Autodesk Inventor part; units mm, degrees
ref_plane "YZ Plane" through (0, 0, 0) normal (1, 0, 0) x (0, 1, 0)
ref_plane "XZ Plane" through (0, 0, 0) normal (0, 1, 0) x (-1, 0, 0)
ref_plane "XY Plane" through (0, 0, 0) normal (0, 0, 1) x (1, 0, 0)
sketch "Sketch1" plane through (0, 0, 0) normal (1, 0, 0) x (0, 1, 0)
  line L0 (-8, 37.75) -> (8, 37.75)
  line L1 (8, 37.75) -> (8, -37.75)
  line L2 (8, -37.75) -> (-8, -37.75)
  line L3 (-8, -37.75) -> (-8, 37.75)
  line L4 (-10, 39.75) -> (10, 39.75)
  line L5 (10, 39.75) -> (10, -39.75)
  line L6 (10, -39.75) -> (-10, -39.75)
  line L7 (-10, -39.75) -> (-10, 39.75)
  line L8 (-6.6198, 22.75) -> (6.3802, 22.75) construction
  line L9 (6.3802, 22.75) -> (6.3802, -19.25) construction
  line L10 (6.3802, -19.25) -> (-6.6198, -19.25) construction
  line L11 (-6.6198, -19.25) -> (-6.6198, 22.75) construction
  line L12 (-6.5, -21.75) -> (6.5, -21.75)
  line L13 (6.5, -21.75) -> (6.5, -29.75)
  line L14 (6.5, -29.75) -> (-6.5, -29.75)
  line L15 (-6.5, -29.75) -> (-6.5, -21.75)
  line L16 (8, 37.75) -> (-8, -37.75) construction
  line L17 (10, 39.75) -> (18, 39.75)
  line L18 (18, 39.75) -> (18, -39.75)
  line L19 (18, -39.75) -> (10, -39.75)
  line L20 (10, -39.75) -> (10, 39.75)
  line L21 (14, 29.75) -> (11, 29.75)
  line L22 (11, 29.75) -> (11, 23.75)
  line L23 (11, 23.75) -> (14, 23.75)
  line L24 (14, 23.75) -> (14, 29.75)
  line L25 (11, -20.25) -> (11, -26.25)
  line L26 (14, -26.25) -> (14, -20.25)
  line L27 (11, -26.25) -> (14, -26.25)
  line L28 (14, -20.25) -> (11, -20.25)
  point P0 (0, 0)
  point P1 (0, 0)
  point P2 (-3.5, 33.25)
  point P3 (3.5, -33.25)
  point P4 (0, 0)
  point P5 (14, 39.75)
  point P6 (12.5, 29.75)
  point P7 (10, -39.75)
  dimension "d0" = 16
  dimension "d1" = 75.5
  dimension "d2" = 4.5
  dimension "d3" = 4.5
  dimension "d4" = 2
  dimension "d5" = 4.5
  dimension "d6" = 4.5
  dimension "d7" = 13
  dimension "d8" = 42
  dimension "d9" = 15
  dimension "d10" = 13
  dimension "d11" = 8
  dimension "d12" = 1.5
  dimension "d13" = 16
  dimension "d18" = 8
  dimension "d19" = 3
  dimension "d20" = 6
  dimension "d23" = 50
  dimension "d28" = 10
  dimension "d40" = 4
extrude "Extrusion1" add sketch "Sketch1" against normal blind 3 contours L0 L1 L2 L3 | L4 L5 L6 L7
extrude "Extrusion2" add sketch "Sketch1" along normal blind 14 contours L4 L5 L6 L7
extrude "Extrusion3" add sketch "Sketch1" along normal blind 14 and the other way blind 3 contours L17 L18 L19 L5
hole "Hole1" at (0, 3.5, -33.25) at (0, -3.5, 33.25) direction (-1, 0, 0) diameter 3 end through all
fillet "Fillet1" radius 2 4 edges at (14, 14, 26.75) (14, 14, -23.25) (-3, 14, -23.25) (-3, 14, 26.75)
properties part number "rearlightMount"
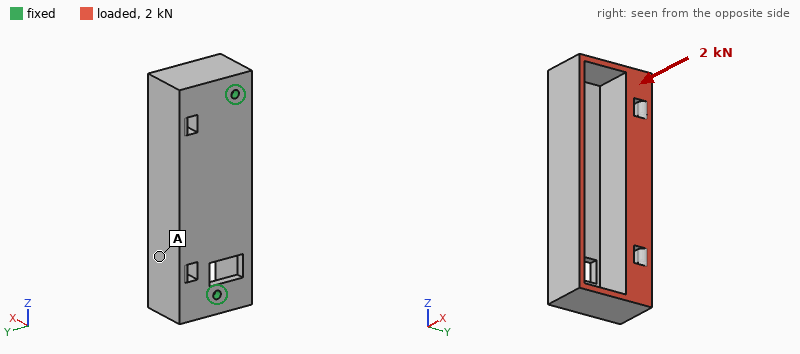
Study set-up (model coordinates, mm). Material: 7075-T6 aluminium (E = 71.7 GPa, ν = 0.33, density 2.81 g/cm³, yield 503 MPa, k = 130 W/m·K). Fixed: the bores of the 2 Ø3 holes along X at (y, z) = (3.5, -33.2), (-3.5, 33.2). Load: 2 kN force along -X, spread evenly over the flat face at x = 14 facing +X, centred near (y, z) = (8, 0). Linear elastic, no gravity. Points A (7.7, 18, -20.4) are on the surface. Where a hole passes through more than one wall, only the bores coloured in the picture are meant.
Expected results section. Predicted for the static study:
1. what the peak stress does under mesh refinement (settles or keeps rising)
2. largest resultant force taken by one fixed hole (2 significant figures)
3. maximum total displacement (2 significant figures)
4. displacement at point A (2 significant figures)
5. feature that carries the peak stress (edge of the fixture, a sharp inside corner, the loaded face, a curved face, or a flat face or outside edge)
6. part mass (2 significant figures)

keeps rising
1.1 kN
0.22 mm
0.13 mm
edge of the fixture
56 g
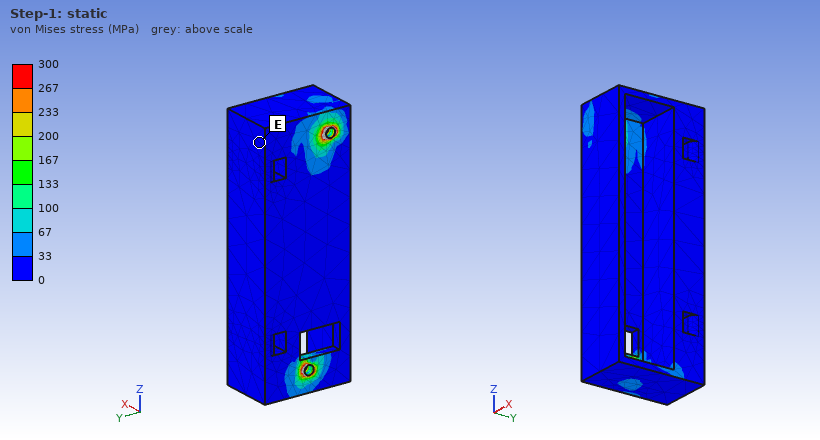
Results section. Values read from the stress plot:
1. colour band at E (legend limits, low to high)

0 to 33 MPa
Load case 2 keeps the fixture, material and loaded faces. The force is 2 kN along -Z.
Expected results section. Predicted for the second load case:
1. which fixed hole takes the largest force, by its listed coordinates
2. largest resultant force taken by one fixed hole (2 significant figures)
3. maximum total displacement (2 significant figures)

(-3.5, 33.2)
1.2 kN
69 µm
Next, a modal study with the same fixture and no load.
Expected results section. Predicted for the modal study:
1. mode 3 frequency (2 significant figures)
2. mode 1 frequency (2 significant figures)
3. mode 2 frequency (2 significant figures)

6700 Hz
2300 Hz
5400 Hz
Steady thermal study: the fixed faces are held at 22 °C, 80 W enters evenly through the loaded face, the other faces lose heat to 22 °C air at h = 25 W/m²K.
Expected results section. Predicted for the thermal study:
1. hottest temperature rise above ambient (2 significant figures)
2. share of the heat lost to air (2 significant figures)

61 K
13 %
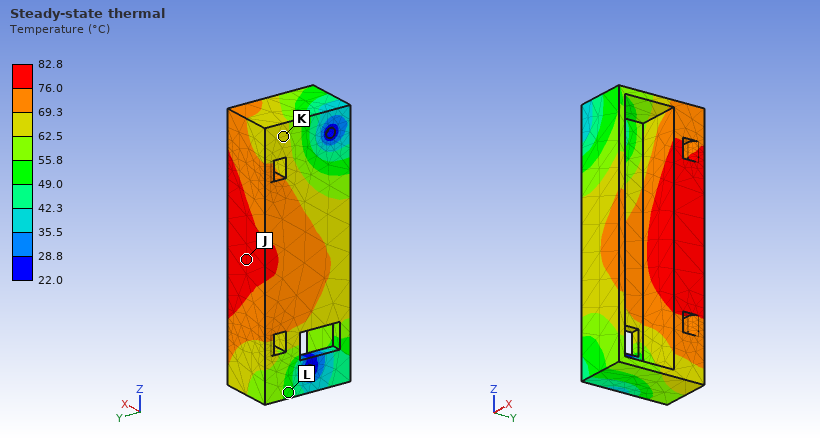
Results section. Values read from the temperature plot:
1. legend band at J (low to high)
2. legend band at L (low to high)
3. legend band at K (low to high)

76.0 to 82.8 °C
49.0 to 55.8 °C
62.5 to 69.3 °C
